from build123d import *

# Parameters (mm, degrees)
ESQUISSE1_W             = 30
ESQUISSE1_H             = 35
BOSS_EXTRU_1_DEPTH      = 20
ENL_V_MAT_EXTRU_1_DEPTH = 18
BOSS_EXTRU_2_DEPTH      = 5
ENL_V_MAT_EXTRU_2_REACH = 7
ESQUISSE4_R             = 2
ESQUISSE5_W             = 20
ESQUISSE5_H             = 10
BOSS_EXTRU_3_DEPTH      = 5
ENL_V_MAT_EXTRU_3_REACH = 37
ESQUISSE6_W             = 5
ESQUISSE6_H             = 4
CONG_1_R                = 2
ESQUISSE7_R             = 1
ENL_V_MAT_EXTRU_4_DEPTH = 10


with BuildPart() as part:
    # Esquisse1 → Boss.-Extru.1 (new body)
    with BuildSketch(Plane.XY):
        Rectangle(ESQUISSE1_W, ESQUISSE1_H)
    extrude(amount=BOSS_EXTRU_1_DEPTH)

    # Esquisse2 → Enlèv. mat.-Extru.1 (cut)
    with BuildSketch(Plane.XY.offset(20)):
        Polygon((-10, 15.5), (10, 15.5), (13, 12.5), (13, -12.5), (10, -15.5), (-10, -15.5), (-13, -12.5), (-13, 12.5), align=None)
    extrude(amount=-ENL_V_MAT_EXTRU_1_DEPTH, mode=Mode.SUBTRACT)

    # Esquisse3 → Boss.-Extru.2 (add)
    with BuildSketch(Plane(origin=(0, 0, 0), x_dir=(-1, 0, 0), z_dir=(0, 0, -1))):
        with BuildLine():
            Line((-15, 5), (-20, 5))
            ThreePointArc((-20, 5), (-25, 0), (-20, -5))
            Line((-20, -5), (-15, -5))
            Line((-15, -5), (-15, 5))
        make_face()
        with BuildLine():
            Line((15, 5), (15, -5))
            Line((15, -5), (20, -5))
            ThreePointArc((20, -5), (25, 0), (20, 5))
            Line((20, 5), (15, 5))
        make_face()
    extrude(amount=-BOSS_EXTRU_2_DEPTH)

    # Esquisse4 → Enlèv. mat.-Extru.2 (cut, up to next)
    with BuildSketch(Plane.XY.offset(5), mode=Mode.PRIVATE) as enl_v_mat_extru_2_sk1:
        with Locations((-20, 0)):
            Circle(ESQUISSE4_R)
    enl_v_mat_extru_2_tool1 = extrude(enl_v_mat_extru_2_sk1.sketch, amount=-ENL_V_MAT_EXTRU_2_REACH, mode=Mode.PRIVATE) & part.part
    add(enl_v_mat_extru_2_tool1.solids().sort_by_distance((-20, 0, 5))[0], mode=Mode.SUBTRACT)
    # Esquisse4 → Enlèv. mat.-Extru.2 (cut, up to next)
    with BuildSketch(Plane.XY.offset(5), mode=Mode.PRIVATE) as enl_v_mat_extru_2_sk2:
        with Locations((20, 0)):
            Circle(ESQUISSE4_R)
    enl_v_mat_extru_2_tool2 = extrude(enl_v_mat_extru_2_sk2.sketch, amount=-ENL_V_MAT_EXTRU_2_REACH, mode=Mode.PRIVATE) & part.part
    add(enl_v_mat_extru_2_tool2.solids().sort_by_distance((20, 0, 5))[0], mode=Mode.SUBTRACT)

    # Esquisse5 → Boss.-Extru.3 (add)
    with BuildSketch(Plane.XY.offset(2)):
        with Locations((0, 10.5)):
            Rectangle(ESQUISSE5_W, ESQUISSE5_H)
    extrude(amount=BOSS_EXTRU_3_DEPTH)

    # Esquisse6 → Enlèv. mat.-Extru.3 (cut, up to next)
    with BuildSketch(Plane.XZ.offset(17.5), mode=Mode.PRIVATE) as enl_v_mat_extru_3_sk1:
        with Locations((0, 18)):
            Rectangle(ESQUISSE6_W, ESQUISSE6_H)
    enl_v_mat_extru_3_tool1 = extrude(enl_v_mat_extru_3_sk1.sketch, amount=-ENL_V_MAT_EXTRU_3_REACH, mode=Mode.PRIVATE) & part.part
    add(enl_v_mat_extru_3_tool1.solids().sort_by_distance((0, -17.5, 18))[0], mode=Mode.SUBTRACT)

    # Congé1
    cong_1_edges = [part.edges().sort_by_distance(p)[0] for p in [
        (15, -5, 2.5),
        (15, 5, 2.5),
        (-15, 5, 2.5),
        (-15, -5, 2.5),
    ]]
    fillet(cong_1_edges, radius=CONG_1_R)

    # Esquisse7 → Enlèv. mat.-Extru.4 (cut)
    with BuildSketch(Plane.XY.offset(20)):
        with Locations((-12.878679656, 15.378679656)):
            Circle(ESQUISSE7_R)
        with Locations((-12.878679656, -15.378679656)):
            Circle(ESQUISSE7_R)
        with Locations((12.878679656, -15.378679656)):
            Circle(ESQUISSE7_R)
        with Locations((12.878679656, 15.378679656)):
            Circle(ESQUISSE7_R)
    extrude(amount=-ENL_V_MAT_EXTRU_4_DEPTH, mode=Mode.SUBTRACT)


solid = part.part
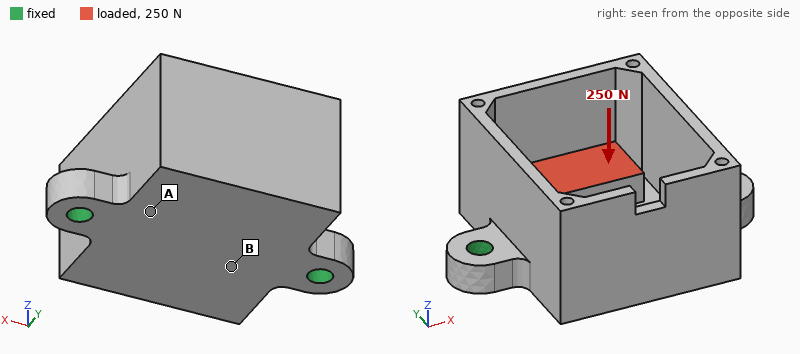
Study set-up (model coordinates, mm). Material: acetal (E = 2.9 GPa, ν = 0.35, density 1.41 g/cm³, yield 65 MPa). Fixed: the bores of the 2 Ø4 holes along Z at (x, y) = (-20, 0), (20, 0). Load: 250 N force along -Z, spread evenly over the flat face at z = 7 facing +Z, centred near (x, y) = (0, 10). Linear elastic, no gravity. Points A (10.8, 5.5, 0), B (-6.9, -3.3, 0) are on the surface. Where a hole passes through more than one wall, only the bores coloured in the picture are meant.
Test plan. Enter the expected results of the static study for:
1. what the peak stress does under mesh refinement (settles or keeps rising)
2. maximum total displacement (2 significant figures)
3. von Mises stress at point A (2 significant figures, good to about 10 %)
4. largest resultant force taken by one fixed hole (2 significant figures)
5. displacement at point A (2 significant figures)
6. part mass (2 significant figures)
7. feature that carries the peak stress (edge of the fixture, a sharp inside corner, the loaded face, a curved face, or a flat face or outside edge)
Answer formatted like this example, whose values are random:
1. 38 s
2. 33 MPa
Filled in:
1. keeps rising
2. 0.57 mm
3. 7.5 MPa
4. 130 N
5. 0.19 mm
6. 12 g
7. edge of the fixture
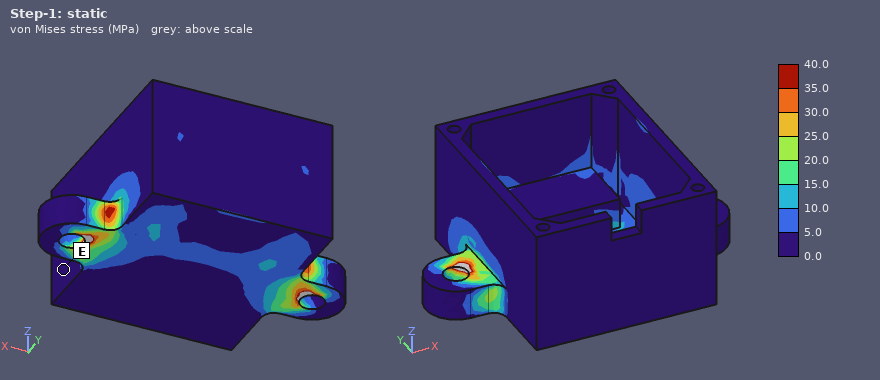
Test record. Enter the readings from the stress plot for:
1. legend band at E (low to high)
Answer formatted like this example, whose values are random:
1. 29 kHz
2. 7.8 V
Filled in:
1. 0.0 to 5.0 MPa
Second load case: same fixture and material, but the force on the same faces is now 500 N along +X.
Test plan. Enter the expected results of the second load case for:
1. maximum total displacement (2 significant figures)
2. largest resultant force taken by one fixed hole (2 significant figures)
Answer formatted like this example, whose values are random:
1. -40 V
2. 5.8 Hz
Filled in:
1. 0.36 mm
2. 300 N
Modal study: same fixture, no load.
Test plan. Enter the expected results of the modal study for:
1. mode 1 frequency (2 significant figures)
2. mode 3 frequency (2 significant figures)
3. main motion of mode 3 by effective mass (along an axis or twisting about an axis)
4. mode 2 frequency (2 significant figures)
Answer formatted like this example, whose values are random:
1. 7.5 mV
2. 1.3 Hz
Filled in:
1. 1200 Hz
2. 2900 Hz
3. along Z
4. 2000 Hz
